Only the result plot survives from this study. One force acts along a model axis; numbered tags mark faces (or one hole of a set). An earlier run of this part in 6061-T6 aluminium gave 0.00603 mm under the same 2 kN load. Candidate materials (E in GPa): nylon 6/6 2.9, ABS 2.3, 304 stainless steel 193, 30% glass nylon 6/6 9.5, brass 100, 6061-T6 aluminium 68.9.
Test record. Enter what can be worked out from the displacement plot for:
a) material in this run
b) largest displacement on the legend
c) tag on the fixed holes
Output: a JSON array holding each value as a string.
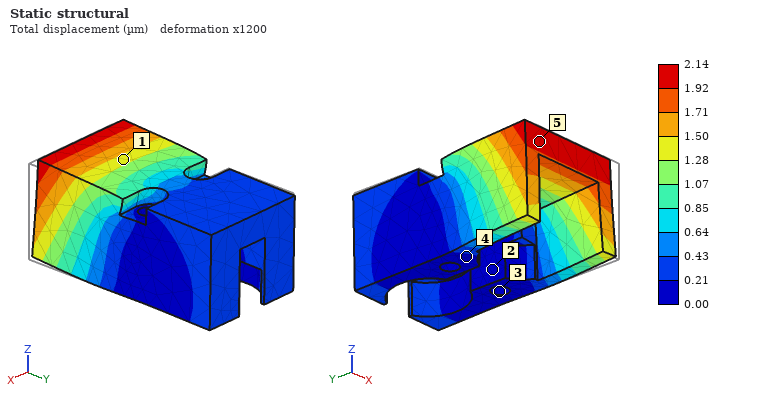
["304 stainless steel", "2.14 µm", "3"]
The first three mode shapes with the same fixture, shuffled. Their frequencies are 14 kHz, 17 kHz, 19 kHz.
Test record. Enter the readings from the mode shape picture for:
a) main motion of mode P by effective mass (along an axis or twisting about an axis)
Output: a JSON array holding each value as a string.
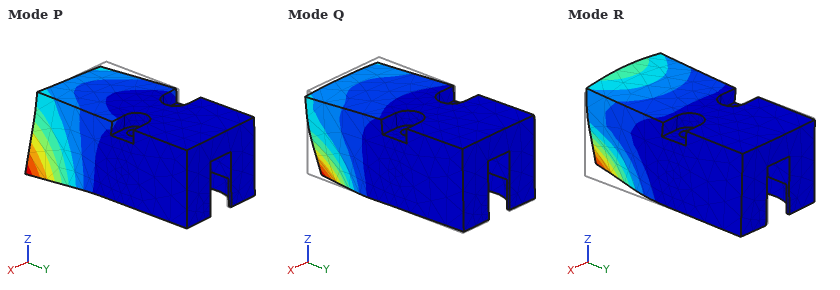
["along X"]
